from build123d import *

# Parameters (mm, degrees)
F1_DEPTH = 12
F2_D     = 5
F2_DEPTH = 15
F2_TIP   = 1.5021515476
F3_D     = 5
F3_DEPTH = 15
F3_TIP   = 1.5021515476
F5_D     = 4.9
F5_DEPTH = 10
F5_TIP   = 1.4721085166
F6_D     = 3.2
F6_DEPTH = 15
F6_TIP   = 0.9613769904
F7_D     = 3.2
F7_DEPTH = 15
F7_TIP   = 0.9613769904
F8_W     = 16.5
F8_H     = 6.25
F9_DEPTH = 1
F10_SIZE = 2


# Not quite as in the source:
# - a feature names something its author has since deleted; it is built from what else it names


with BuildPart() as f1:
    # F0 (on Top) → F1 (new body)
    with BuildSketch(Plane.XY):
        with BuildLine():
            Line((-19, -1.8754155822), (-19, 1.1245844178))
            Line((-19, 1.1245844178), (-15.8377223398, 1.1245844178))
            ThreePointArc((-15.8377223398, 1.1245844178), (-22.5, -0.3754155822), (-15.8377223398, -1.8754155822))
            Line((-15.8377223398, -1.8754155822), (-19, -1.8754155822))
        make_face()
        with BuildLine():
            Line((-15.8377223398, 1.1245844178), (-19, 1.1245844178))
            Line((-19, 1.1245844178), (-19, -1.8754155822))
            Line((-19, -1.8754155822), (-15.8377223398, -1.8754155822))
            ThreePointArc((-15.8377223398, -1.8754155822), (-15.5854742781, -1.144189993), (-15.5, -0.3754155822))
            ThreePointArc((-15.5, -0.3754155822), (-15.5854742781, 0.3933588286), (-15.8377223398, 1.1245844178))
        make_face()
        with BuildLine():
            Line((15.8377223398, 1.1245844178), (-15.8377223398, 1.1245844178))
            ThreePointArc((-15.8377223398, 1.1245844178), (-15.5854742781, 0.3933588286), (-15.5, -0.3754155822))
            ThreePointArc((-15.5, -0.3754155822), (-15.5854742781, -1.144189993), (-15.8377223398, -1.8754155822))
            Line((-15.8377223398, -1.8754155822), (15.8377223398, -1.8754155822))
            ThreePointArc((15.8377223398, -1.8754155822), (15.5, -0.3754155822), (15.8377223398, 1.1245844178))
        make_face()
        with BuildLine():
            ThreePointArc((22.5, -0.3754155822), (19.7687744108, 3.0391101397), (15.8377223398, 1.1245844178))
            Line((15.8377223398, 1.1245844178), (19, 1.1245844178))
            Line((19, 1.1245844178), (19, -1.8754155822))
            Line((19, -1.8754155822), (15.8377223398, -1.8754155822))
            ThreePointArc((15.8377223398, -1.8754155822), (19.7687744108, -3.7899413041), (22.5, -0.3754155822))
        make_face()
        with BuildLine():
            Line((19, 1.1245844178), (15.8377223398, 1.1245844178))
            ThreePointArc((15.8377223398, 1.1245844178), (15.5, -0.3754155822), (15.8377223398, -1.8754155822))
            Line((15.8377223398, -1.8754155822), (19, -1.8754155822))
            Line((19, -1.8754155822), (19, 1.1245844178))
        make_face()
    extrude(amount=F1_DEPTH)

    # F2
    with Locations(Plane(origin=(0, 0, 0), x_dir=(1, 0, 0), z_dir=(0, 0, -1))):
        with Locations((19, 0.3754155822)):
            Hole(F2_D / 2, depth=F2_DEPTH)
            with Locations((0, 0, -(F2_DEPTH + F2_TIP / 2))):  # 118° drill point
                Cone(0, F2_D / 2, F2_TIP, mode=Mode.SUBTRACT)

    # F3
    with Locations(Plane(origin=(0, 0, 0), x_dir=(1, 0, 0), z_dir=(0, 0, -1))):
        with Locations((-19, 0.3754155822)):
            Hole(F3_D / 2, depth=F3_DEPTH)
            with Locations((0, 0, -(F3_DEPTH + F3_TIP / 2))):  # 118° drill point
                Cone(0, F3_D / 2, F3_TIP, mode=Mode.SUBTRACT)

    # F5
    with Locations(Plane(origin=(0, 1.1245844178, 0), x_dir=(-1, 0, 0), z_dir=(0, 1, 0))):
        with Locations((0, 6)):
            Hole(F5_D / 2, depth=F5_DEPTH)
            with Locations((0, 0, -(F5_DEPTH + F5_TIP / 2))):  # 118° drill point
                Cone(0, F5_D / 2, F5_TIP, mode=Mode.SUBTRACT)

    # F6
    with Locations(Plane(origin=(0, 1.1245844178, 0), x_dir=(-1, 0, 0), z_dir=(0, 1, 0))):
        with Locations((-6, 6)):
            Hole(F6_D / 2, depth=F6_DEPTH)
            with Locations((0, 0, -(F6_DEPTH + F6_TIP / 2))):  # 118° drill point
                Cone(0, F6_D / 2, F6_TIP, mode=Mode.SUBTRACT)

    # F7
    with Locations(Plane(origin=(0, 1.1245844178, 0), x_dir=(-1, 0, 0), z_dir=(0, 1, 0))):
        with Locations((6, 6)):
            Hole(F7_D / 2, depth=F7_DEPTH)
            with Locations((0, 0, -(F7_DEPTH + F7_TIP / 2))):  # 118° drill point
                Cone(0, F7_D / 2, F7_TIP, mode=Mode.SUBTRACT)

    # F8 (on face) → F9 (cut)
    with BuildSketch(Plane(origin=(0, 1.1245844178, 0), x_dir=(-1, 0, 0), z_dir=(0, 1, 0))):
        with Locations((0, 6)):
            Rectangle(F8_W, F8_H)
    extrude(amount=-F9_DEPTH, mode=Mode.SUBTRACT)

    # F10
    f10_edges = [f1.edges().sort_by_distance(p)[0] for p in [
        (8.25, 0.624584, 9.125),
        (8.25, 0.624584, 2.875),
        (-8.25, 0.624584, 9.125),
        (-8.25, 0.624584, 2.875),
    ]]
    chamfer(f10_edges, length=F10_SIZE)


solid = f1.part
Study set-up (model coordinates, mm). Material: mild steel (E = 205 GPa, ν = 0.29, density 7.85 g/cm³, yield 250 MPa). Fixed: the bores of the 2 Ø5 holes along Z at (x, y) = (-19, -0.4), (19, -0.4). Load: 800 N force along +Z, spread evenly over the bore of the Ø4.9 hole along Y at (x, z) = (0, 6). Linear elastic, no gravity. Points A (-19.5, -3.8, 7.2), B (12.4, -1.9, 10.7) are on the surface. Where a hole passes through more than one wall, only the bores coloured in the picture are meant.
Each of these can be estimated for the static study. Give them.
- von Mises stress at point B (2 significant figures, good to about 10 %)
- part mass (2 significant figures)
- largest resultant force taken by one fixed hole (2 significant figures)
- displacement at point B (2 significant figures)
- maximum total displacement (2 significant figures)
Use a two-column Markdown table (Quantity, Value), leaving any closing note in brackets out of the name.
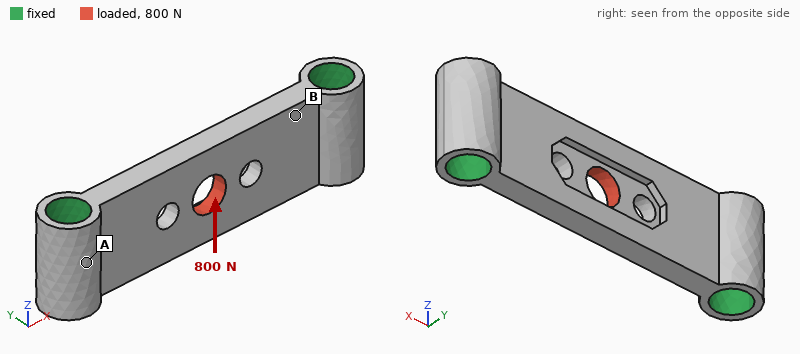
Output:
| Quantity | Value |
|---|---|
| von Mises stress at point B | 23 MPa |
| part mass | 11 g |
| largest resultant force taken by one fixed hole | 400 N |
| displacement at point B | 1.1 µm |
| maximum total displacement | 6.1 µm |
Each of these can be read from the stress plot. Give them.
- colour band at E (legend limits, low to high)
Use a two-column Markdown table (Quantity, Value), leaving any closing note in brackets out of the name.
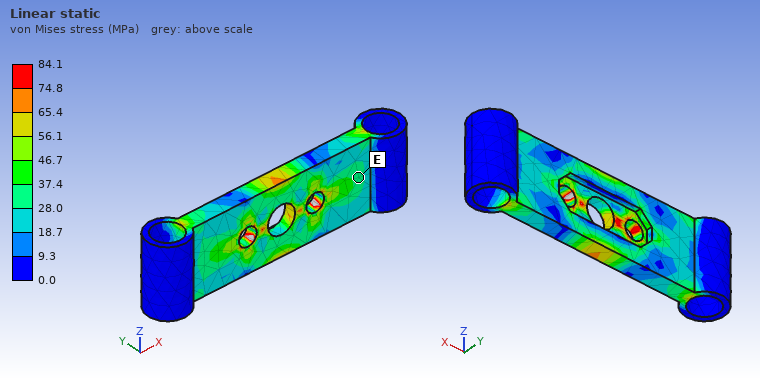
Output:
| Quantity | Value |
|---|---|
| colour band at E | 28.0 to 37.4 MPa |
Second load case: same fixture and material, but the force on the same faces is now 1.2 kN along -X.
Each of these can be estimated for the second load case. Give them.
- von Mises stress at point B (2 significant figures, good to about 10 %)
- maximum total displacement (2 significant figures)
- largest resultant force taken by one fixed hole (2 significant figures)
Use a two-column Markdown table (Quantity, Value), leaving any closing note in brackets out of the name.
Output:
| Quantity | Value |
|---|---|
| von Mises stress at point B | 20 MPa |
| maximum total displacement | 2.4 µm |
| largest resultant force taken by one fixed hole | 600 N |
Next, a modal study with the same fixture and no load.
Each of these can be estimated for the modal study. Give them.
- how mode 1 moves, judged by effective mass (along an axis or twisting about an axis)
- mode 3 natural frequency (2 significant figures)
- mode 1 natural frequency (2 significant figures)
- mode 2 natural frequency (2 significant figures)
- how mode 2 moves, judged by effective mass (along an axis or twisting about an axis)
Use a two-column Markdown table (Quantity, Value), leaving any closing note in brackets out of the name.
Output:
| Quantity | Value |
|---|---|
| how mode 1 moves, judged by effective mass | along Y |
| mode 3 natural frequency | 35 kHz |
| mode 1 natural frequency | 15 kHz |
| mode 2 natural frequency | 24 kHz |
| how mode 2 moves, judged by effective mass | twisting about X |
